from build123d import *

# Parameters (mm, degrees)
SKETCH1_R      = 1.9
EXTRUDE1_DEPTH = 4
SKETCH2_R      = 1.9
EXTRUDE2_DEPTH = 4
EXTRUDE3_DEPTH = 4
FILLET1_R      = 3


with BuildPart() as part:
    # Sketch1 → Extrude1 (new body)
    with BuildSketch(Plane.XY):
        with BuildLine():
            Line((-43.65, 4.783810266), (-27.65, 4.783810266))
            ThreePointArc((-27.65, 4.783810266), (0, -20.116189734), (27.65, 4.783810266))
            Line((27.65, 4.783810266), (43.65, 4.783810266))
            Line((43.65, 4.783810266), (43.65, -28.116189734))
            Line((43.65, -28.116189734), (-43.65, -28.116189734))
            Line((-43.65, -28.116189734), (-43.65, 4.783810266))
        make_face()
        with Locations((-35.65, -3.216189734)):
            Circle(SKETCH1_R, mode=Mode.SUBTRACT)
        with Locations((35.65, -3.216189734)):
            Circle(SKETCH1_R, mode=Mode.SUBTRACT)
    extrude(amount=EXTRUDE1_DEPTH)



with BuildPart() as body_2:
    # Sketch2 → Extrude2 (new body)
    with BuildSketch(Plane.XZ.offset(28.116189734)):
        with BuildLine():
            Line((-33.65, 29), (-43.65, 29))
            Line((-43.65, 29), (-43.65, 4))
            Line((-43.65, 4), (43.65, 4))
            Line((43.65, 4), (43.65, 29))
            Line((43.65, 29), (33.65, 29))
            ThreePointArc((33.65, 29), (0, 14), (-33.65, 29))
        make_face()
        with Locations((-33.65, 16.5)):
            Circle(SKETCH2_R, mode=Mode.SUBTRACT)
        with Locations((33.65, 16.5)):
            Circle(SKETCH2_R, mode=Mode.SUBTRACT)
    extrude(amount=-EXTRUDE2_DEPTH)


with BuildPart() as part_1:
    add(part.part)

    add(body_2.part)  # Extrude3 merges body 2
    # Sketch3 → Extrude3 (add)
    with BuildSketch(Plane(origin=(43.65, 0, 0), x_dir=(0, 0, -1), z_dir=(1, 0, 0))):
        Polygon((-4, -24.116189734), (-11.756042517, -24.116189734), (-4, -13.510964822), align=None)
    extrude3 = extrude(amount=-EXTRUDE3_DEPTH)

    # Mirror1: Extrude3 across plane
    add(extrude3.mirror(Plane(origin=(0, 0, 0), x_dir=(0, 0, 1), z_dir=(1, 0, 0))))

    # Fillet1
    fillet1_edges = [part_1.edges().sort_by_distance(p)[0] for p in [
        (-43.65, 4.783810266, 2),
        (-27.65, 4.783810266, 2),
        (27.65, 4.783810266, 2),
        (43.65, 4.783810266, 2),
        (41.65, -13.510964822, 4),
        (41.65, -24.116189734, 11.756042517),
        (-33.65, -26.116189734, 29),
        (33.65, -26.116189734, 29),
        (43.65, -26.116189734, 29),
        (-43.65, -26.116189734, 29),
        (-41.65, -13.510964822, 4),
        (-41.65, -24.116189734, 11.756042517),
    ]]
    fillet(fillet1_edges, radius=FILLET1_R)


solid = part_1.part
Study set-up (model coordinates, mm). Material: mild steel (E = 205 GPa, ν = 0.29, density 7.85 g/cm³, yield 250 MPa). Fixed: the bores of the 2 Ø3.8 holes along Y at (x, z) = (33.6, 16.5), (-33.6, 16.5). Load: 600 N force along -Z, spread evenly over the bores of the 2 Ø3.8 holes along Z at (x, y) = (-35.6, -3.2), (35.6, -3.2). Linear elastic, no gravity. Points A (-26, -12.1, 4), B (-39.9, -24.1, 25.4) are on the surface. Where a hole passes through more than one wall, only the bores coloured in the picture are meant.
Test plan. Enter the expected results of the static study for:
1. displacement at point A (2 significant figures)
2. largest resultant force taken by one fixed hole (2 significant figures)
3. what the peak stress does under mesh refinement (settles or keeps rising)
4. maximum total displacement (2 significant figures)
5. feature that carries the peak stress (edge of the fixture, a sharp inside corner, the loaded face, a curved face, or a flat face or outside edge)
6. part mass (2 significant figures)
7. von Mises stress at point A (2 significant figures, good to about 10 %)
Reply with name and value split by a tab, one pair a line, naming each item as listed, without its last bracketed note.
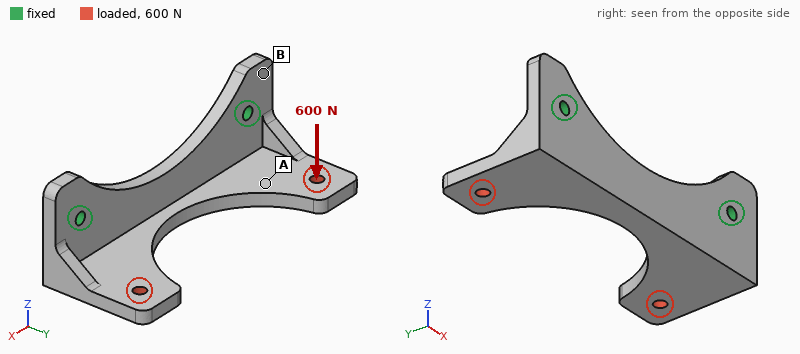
displacement at point A	0.048 mm
largest resultant force taken by one fixed hole	300 N
what the peak stress does under mesh refinement	keeps rising
maximum total displacement	0.13 mm
feature that carries the peak stress	edge of the fixture
part mass	100 g
von Mises stress at point A	39 MPa
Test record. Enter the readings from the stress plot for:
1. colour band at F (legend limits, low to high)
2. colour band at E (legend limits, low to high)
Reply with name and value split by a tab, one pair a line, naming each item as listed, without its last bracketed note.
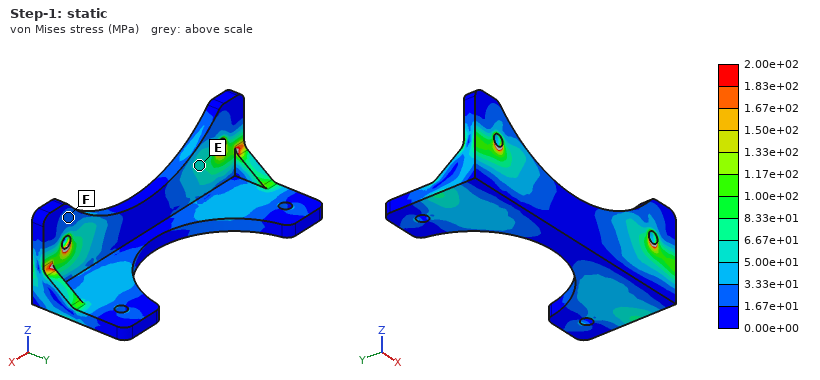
colour band at F	1.67e+01 to 3.33e+01 MPa
colour band at E	5.00e+01 to 6.67e+01 MPa
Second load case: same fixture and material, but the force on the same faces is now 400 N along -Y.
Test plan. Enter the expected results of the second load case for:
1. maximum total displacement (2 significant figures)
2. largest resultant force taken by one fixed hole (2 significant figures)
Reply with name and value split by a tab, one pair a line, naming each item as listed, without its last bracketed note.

maximum total displacement	27 µm
largest resultant force taken by one fixed hole	200 N
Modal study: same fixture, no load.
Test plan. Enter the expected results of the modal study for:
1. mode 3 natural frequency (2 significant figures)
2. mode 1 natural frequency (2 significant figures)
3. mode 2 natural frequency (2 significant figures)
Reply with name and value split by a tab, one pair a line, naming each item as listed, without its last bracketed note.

mode 3 natural frequency	4100 Hz
mode 1 natural frequency	2500 Hz
mode 2 natural frequency	3000 Hz
